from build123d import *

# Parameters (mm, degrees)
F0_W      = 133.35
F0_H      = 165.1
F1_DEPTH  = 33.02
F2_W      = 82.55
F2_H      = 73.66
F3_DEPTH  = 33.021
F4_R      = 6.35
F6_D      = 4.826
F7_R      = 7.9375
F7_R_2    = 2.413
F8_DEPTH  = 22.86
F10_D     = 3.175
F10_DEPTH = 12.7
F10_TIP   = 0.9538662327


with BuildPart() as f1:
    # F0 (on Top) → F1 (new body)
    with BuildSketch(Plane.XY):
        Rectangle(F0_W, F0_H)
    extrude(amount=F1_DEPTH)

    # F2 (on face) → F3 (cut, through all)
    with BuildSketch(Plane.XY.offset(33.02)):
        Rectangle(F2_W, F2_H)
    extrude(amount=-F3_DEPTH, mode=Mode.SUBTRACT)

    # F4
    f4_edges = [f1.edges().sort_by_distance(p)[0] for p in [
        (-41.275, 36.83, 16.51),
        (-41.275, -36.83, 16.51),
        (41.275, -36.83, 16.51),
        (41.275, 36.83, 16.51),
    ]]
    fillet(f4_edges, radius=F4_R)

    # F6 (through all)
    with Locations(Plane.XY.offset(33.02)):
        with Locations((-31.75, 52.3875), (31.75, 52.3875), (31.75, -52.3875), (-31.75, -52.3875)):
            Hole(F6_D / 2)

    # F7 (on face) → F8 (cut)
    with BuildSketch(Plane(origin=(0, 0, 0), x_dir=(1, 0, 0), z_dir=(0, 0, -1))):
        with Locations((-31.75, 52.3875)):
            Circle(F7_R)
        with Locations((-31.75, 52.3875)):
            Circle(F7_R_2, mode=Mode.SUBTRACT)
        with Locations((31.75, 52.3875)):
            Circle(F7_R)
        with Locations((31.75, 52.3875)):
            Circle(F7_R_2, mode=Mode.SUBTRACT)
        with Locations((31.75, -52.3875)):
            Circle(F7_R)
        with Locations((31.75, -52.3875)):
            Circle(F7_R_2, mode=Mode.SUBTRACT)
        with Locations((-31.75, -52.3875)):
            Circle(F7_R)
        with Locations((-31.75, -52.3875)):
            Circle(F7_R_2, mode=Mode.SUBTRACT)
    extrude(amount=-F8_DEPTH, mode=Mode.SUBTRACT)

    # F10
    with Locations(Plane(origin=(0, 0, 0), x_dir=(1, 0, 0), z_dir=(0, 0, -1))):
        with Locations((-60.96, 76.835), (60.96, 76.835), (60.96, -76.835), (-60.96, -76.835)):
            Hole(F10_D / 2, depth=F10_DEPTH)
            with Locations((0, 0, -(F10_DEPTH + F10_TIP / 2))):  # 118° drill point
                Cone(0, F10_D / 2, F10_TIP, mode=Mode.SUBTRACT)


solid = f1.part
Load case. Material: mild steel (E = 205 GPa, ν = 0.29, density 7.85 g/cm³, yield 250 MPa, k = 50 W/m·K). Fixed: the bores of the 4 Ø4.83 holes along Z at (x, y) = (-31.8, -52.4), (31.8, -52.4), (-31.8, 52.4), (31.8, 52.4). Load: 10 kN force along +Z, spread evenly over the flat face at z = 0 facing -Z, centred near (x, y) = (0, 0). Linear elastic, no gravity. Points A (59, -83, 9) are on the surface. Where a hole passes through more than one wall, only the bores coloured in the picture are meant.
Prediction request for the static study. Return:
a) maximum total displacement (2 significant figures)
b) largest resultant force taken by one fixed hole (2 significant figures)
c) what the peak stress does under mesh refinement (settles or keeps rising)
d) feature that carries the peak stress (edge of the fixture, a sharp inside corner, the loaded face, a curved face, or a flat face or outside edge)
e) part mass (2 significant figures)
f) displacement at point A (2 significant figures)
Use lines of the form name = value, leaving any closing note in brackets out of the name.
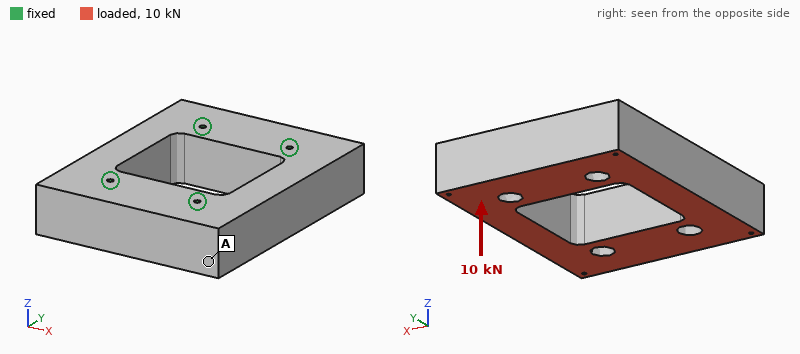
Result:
maximum total displacement = 3.1 µm
largest resultant force taken by one fixed hole = 2.6 kN
what the peak stress does under mesh refinement = keeps rising
feature that carries the peak stress = edge of the fixture
part mass = 4.0 kg
displacement at point A = 2.1 µm
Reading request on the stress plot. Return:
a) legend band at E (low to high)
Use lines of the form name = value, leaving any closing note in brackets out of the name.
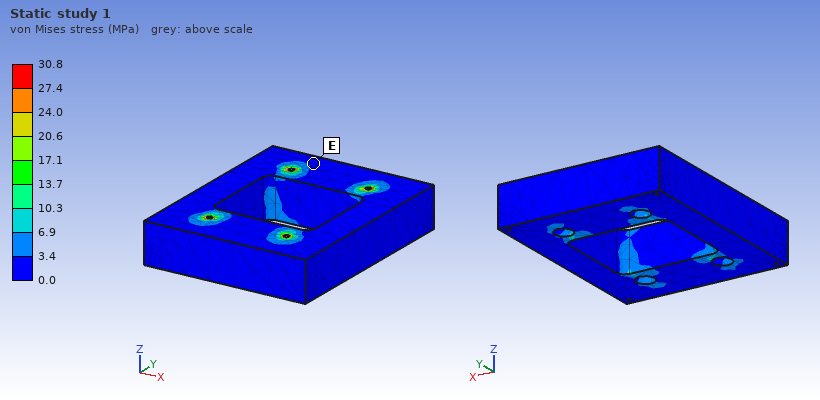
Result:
legend band at E = 0.0 to 3.4 MPa
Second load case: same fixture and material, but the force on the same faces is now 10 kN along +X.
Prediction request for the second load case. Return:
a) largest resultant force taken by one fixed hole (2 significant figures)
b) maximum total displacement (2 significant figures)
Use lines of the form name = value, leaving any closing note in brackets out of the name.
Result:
largest resultant force taken by one fixed hole = 3.3 kN
maximum total displacement = 5.8 µm
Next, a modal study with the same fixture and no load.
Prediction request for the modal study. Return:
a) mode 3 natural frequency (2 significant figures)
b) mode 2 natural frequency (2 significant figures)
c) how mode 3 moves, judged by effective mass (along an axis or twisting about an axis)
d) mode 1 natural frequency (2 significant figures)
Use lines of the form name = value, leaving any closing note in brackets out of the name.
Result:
mode 3 natural frequency = 5000 Hz
mode 2 natural frequency = 4800 Hz
how mode 3 moves, judged by effective mass = along Y
mode 1 natural frequency = 4400 Hz
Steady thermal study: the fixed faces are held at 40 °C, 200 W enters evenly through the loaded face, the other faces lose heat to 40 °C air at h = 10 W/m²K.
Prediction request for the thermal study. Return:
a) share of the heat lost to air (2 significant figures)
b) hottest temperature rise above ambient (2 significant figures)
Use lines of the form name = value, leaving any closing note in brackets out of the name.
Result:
share of the heat lost to air = 7.8 %
hottest temperature rise above ambient = 41 K
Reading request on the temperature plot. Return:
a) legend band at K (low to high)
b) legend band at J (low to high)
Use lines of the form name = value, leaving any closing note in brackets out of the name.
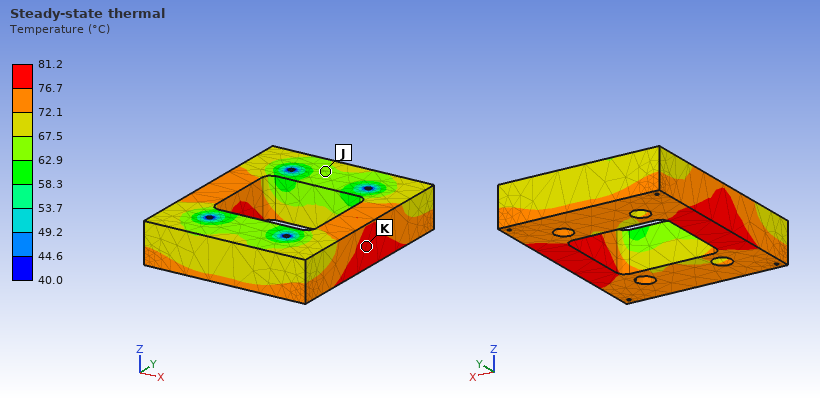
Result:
legend band at K = 76.7 to 81.2 °C
legend band at J = 62.9 to 67.5 °C
